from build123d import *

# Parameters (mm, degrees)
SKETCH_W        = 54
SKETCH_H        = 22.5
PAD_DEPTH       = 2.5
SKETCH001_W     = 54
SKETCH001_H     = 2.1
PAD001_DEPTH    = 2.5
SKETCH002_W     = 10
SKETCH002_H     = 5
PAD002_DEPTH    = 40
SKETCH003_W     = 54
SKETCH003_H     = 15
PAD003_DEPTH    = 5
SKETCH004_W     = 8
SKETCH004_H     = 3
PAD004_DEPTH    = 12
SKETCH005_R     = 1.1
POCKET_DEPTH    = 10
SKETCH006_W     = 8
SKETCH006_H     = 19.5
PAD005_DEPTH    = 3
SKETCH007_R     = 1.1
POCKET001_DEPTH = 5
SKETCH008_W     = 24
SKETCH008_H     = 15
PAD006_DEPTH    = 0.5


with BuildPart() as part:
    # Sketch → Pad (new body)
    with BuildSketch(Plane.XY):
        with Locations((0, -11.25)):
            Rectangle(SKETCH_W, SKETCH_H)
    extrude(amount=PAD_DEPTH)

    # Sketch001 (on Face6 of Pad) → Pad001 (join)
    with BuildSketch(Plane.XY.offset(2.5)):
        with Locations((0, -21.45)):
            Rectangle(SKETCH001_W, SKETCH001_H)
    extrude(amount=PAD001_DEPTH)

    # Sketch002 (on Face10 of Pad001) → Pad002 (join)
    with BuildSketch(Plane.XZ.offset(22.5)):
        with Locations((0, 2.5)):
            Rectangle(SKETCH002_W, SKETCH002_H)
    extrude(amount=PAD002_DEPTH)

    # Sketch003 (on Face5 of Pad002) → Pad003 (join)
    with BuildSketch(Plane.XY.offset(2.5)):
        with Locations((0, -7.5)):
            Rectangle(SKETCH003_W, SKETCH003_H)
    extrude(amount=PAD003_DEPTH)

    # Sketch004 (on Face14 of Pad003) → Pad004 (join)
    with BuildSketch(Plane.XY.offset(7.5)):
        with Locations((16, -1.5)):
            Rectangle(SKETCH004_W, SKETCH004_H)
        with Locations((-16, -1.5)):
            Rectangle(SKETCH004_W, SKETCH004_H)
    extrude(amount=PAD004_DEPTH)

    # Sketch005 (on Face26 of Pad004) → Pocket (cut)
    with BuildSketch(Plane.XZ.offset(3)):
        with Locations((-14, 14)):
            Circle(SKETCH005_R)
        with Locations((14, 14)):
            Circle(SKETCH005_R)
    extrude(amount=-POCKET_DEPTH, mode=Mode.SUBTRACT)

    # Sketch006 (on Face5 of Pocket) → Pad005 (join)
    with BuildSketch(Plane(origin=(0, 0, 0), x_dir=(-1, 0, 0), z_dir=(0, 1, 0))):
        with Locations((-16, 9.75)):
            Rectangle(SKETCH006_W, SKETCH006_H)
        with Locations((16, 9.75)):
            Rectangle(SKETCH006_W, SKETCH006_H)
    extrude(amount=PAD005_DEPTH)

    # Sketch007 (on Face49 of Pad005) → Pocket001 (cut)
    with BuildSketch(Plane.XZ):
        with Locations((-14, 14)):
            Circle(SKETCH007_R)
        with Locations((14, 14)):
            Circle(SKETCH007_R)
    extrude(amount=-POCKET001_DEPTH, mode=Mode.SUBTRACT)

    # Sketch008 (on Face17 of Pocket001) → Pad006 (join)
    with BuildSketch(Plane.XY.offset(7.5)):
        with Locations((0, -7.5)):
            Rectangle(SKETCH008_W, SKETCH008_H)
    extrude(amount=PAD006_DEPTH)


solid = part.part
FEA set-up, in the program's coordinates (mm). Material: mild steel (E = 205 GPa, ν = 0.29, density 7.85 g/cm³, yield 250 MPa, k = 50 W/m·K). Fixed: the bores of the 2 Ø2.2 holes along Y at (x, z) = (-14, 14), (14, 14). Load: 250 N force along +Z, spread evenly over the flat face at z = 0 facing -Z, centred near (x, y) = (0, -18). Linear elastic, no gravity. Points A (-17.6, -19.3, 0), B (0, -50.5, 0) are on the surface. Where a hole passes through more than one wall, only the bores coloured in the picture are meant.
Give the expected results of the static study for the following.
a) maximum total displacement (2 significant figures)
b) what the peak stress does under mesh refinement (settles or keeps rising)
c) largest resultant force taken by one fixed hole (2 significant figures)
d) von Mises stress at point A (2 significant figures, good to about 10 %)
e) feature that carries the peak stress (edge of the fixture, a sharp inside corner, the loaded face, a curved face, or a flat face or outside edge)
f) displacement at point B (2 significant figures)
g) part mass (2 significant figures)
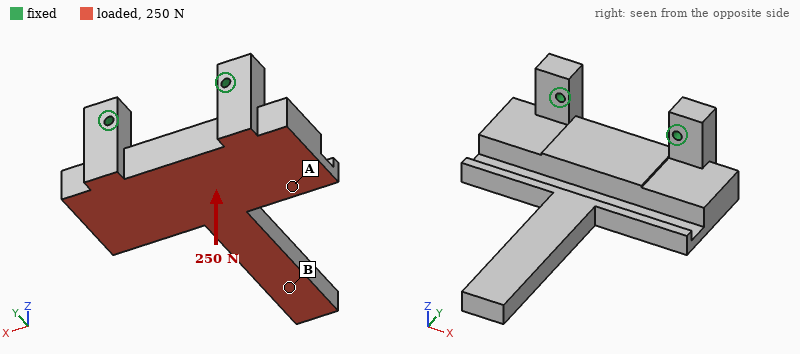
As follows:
0.15 mm
keeps rising
130 N
16 MPa
edge of the fixture
0.11 mm
86 g
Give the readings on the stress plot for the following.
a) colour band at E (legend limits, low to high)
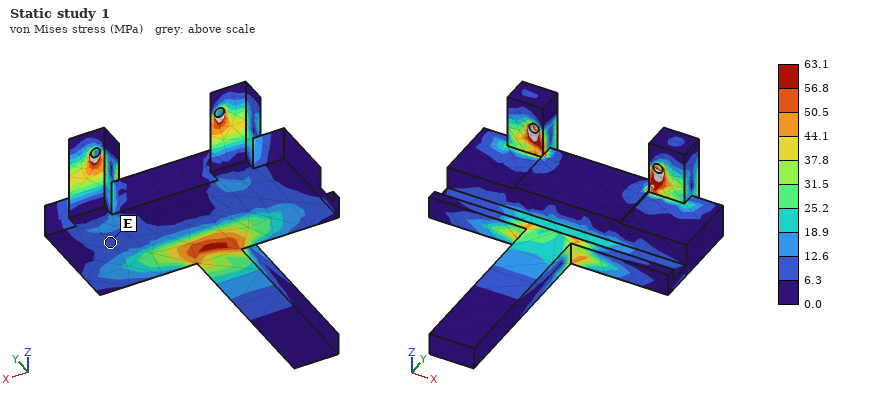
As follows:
6.3 to 12.6 MPa
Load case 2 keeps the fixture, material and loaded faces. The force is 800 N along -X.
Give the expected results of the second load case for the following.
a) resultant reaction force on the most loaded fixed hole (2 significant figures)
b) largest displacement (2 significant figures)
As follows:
660 N
49 µm
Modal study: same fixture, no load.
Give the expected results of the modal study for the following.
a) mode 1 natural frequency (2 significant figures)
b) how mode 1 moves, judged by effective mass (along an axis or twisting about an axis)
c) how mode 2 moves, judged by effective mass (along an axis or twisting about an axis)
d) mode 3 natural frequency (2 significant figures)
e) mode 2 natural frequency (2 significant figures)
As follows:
1100 Hz
along Z
along X
3900 Hz
3300 Hz
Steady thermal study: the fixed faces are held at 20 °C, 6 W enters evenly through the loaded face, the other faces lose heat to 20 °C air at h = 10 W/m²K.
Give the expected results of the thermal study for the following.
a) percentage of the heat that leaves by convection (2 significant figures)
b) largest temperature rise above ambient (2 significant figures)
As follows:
9.7 %
29 K
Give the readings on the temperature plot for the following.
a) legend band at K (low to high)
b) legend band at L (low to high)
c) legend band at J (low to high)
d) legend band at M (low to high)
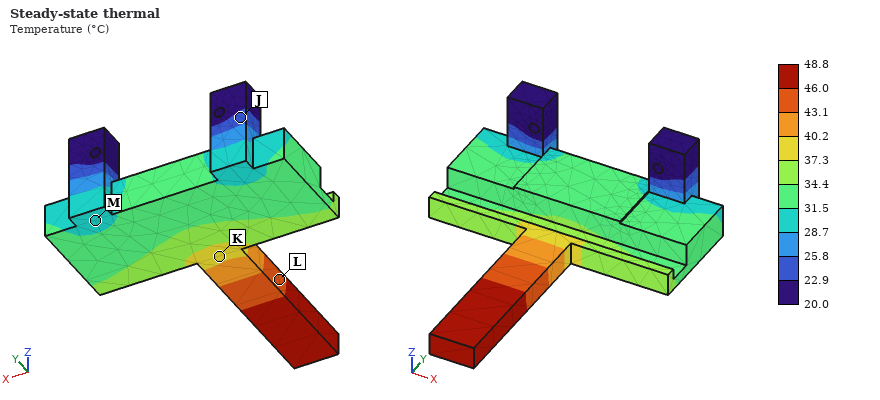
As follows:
37.3 to 40.2 °C
43.1 to 46.0 °C
22.9 to 25.8 °C
28.7 to 31.5 °C
